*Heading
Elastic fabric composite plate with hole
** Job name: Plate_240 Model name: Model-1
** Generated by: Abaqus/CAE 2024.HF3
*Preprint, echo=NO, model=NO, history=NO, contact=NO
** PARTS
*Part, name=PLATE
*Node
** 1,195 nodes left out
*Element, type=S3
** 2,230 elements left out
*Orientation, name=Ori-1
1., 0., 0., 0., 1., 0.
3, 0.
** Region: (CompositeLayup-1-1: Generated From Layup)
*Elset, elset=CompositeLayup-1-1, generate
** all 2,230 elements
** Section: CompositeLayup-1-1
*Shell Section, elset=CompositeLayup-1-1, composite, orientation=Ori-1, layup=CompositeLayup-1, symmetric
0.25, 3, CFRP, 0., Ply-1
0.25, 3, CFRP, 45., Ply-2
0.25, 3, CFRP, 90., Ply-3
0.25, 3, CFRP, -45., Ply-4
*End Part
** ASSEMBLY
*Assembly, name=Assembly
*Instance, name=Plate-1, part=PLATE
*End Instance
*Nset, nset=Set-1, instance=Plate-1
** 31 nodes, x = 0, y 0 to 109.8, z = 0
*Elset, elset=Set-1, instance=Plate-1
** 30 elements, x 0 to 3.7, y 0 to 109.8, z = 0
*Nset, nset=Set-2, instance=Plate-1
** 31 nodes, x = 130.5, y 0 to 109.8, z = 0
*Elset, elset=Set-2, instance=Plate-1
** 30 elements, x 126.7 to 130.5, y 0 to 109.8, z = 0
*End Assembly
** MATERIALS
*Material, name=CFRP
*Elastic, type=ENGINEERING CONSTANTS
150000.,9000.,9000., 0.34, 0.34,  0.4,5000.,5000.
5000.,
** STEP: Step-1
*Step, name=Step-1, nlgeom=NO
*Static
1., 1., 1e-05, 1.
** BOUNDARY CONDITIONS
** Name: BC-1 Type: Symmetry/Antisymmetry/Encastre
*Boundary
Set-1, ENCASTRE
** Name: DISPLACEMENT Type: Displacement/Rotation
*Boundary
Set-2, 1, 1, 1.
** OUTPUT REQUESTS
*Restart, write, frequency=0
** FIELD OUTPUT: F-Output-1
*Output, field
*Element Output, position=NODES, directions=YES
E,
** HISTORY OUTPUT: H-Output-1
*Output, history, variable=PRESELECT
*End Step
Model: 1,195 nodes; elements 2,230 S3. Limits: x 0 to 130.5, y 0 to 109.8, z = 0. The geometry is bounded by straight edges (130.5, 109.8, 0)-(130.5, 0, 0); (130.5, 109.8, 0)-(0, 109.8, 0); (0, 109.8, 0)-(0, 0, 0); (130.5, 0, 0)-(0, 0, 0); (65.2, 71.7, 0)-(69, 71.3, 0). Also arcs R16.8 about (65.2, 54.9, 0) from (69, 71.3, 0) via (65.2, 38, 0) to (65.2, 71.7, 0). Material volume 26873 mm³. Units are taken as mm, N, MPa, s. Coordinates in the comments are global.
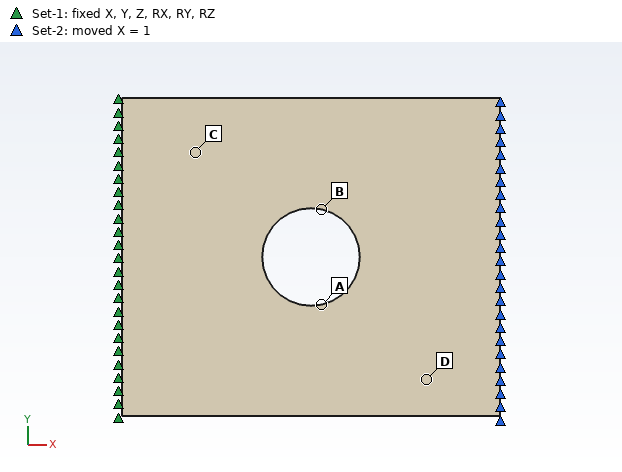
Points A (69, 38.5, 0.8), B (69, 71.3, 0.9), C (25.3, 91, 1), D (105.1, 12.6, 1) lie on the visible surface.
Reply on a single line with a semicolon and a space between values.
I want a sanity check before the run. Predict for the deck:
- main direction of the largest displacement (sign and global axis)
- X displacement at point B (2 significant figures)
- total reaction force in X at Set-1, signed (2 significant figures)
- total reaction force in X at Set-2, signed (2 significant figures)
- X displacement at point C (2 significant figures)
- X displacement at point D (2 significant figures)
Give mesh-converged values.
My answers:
+X; 0.58 mm; -80000 N; 80000 N; 0.18 mm; 0.81 mm
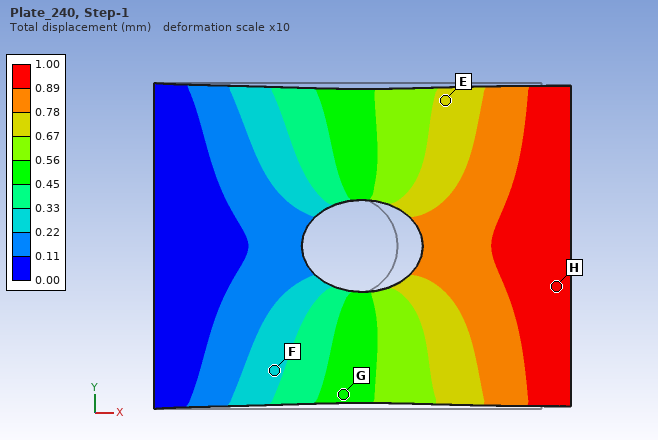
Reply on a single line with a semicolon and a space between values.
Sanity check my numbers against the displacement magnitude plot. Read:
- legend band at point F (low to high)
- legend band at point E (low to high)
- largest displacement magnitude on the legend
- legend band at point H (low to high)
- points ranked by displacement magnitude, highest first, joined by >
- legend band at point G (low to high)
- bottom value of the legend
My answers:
0.22 to 0.33 mm; 0.67 to 0.78 mm; 1.00 mm; 0.89 to 1.00 mm; H > E > G > F; 0.45 to 0.56 mm; 0.00 mm
